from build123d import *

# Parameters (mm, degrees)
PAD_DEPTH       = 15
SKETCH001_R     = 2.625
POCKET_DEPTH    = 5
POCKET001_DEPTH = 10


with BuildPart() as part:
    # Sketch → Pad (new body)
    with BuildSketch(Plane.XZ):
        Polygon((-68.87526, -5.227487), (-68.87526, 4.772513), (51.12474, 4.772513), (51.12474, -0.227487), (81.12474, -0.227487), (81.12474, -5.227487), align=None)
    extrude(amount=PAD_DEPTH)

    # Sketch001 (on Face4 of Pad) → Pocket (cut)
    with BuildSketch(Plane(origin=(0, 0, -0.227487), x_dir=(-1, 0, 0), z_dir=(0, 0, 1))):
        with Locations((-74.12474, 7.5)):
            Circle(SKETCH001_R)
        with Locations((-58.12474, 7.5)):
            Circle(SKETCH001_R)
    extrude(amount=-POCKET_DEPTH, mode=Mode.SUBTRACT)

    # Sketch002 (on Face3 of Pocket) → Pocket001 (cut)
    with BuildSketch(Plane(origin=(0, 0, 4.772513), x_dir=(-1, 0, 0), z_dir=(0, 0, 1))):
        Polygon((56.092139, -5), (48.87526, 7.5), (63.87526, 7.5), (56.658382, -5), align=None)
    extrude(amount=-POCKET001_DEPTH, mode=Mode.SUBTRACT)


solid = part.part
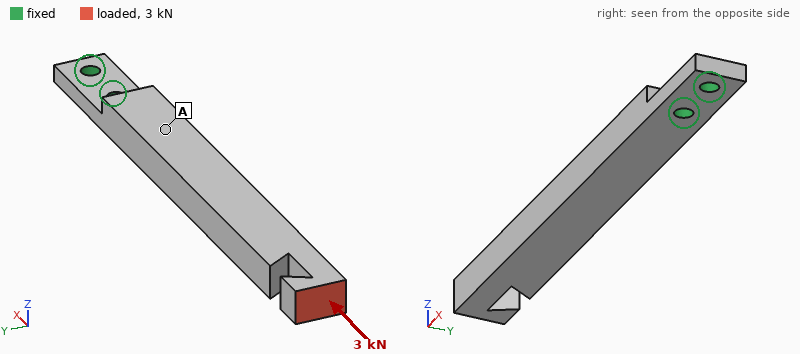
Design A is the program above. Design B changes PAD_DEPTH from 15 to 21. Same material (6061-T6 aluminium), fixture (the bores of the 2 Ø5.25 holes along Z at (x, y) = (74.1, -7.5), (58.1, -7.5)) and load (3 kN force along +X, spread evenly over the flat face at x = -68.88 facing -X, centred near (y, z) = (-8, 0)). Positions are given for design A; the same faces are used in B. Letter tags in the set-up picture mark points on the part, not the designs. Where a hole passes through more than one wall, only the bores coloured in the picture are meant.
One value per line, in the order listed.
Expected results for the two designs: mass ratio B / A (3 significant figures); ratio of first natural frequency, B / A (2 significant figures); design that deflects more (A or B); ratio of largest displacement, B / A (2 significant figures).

1.42
0.95
A
0.74
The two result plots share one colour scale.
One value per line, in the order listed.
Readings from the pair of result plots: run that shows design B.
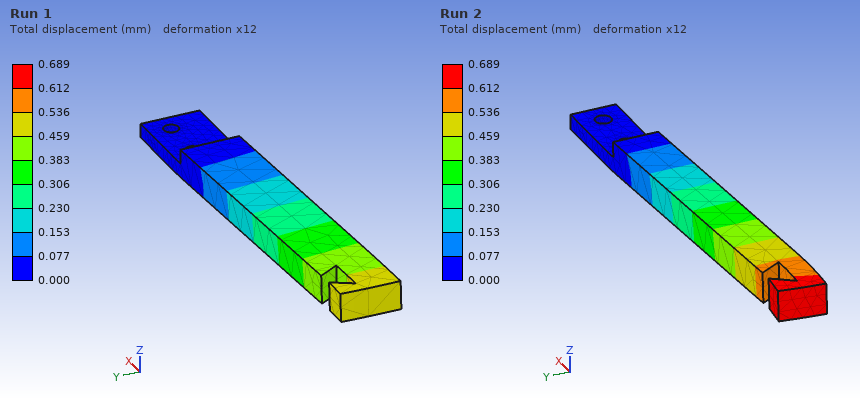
Run 1
